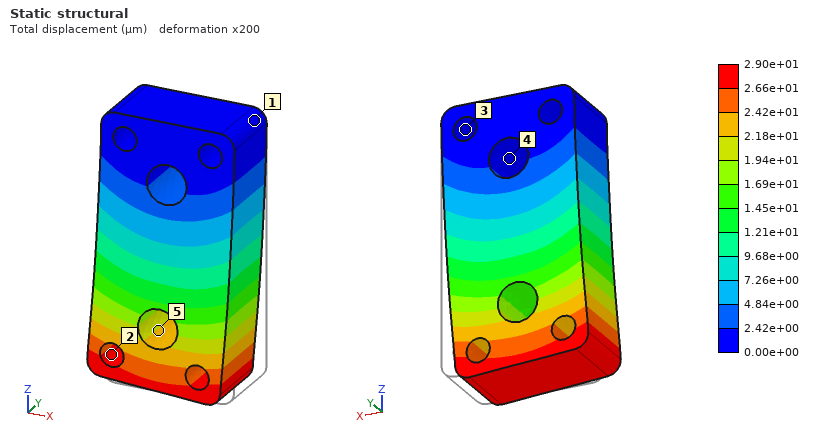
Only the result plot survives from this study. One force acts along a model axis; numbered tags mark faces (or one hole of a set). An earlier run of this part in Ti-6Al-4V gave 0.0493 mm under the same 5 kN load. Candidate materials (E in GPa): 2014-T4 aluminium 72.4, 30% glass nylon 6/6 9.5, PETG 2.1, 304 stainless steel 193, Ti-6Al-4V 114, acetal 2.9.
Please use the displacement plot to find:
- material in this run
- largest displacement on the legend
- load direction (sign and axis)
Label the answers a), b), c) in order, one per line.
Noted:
a) 304 stainless steel
b) 2.90e+01 µm
c) -X
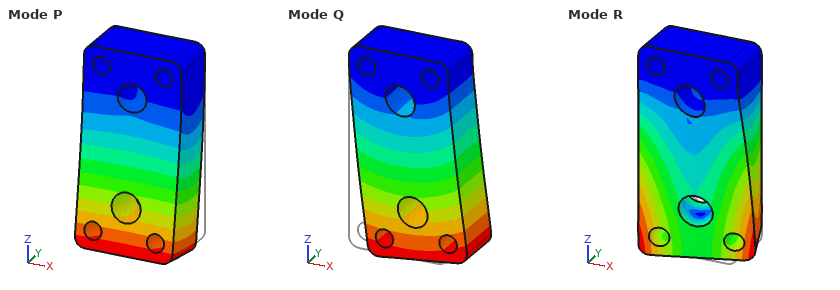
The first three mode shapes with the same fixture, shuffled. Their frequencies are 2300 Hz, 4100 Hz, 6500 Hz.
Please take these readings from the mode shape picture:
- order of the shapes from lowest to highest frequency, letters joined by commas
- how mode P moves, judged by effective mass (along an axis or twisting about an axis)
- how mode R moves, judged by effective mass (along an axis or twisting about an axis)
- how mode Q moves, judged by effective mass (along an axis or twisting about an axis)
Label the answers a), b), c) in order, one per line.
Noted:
a) P, Q, R
b) along Y
c) twisting about Z
d) along X
